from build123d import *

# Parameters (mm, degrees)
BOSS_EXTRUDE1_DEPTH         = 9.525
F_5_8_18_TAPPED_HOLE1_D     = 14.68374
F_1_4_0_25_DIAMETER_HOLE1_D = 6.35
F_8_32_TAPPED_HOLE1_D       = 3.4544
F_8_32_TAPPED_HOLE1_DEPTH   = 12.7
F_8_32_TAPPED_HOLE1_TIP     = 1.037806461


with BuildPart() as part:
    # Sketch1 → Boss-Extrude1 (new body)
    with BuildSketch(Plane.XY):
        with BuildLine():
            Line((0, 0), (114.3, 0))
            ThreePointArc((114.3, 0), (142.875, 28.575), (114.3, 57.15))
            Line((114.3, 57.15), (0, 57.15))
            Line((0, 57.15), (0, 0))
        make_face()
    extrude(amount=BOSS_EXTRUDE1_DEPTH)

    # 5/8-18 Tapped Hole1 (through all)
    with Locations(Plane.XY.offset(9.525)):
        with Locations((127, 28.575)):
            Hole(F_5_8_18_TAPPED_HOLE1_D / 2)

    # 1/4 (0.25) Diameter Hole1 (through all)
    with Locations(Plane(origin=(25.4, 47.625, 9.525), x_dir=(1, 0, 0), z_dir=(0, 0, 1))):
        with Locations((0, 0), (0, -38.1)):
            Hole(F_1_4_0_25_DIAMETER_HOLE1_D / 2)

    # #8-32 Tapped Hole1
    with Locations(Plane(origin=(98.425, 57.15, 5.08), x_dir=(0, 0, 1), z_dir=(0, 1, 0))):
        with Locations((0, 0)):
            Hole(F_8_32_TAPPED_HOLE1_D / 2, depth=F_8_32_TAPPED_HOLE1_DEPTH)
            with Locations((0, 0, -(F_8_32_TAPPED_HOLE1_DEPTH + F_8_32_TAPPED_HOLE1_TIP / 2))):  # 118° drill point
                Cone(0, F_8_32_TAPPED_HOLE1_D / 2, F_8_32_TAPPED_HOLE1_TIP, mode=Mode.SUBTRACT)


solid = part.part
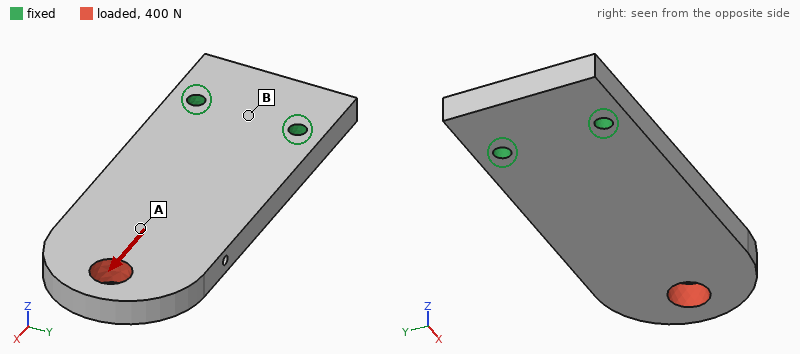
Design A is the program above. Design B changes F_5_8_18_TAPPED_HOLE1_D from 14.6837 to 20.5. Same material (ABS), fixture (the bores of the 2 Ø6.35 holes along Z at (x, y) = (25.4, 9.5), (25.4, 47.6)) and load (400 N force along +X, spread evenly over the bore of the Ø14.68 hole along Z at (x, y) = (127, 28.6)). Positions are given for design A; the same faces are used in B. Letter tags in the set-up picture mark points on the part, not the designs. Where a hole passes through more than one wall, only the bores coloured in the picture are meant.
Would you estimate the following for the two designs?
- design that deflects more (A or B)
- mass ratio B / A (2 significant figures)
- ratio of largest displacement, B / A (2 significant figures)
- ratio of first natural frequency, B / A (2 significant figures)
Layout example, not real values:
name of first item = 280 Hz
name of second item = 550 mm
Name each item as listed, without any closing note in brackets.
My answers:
design that deflects more = B
mass ratio B / A = 0.98
ratio of largest displacement, B / A = 1.2
ratio of first natural frequency, B / A = 1.0
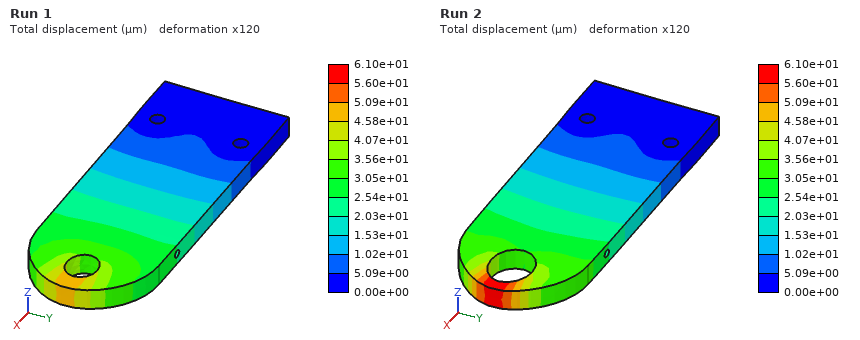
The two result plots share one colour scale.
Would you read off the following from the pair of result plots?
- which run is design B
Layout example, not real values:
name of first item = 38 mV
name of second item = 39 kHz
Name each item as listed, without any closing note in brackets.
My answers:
which run is design B = Run 2
